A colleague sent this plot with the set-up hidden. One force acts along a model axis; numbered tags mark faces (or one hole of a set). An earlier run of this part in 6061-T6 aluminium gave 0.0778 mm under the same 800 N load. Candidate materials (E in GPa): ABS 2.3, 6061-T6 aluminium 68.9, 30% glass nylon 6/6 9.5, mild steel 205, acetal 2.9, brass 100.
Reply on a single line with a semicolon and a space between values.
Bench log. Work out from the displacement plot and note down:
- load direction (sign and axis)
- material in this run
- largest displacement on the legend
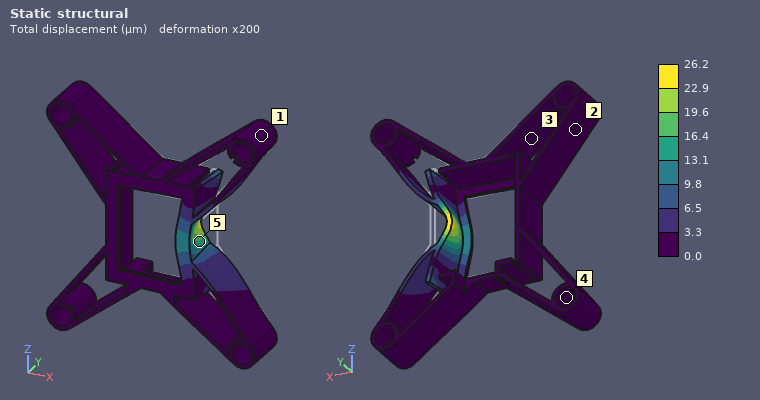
-X; mild steel; 26.2 µm
